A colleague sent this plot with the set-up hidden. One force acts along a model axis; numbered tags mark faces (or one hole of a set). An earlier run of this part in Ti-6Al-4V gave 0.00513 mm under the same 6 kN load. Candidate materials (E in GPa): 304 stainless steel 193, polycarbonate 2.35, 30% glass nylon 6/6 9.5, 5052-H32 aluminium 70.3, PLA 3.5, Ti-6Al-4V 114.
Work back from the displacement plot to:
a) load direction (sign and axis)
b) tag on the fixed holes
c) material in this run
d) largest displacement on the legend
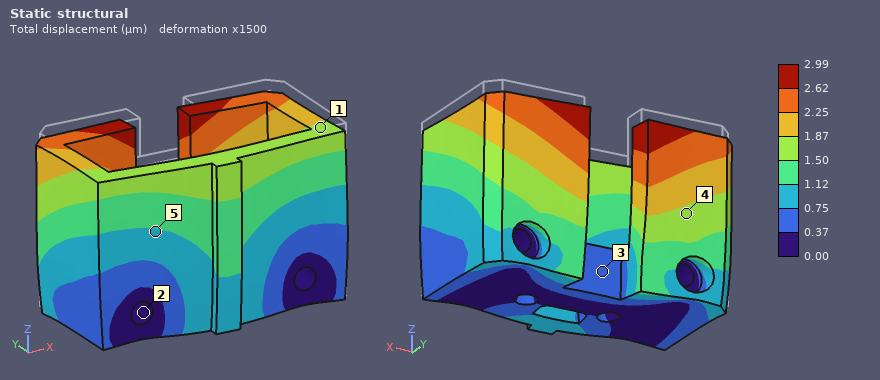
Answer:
-Z
2
304 stainless steel
2.99 µm
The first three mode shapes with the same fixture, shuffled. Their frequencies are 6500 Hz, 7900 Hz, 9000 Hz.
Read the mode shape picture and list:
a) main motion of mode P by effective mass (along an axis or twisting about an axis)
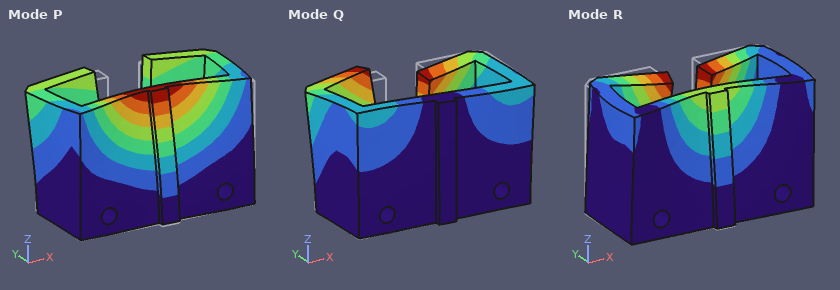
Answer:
along Y
